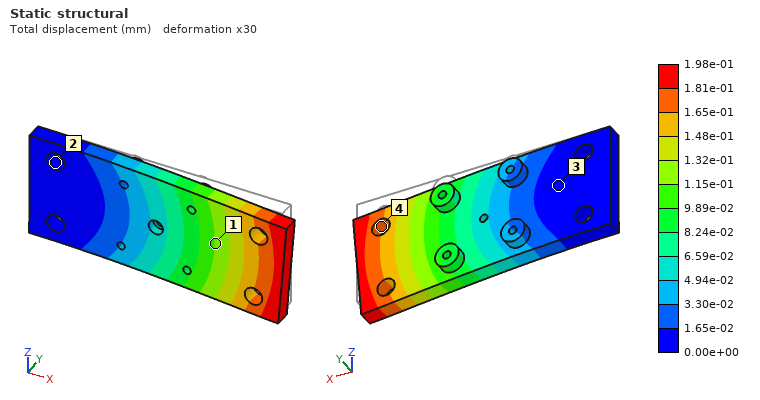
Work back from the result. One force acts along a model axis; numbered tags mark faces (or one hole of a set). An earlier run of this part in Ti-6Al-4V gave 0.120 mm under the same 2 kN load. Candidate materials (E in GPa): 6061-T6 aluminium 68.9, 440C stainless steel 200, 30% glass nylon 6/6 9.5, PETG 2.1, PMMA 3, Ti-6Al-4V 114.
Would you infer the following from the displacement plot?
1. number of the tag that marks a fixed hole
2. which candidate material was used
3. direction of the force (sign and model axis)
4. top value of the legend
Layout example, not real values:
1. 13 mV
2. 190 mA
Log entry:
1. 2
2. 6061-T6 aluminium
3. -Z
4. 1.98e-01 mm
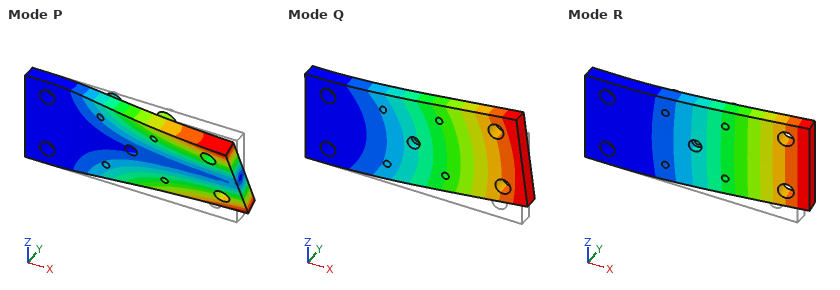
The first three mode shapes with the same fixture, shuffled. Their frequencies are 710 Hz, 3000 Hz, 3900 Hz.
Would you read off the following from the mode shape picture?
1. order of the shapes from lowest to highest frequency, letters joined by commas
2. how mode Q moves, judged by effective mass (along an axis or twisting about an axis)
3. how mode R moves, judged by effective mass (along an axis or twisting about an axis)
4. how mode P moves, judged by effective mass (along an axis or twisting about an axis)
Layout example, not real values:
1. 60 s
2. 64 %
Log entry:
1. R, P, Q
2. along Z
3. along Y
4. twisting about X
